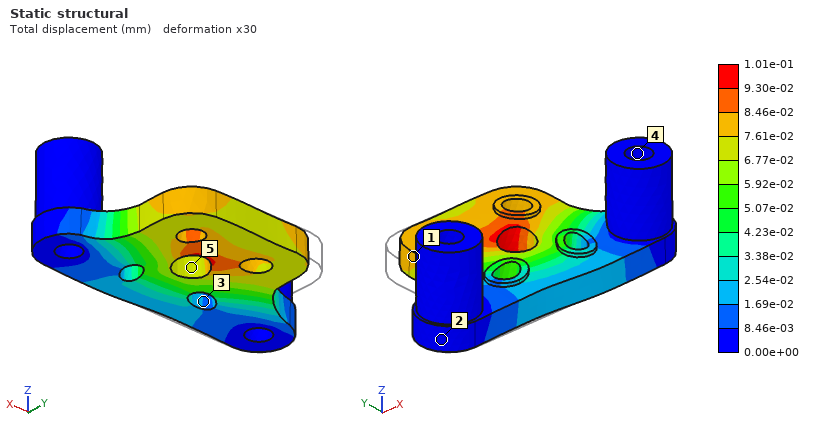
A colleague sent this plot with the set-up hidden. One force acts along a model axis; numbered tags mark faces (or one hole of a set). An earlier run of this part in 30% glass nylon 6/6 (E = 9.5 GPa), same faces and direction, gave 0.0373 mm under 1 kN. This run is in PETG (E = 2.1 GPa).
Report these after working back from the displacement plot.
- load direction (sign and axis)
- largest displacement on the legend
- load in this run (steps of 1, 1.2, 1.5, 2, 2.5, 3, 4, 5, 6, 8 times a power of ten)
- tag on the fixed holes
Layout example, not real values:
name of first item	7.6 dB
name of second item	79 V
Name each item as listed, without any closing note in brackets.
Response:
load direction	+X
largest displacement on the legend	1.01e-01 mm
load in this run	600 N
tag on the fixed holes	4
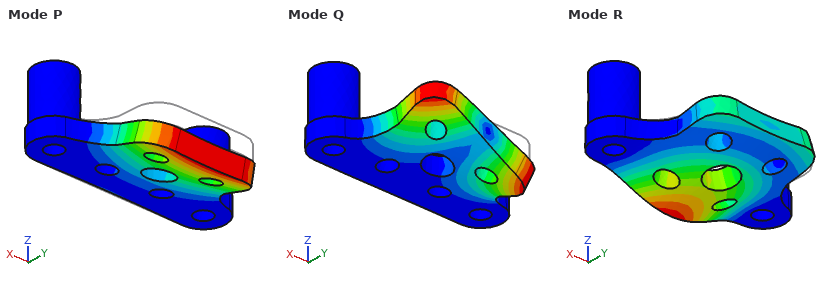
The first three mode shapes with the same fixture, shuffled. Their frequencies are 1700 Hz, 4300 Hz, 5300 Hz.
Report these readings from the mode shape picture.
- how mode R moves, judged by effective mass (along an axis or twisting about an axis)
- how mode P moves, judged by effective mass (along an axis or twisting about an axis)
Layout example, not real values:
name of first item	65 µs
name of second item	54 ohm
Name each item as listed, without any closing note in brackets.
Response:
how mode R moves, judged by effective mass	along Z
how mode P moves, judged by effective mass	along Z
